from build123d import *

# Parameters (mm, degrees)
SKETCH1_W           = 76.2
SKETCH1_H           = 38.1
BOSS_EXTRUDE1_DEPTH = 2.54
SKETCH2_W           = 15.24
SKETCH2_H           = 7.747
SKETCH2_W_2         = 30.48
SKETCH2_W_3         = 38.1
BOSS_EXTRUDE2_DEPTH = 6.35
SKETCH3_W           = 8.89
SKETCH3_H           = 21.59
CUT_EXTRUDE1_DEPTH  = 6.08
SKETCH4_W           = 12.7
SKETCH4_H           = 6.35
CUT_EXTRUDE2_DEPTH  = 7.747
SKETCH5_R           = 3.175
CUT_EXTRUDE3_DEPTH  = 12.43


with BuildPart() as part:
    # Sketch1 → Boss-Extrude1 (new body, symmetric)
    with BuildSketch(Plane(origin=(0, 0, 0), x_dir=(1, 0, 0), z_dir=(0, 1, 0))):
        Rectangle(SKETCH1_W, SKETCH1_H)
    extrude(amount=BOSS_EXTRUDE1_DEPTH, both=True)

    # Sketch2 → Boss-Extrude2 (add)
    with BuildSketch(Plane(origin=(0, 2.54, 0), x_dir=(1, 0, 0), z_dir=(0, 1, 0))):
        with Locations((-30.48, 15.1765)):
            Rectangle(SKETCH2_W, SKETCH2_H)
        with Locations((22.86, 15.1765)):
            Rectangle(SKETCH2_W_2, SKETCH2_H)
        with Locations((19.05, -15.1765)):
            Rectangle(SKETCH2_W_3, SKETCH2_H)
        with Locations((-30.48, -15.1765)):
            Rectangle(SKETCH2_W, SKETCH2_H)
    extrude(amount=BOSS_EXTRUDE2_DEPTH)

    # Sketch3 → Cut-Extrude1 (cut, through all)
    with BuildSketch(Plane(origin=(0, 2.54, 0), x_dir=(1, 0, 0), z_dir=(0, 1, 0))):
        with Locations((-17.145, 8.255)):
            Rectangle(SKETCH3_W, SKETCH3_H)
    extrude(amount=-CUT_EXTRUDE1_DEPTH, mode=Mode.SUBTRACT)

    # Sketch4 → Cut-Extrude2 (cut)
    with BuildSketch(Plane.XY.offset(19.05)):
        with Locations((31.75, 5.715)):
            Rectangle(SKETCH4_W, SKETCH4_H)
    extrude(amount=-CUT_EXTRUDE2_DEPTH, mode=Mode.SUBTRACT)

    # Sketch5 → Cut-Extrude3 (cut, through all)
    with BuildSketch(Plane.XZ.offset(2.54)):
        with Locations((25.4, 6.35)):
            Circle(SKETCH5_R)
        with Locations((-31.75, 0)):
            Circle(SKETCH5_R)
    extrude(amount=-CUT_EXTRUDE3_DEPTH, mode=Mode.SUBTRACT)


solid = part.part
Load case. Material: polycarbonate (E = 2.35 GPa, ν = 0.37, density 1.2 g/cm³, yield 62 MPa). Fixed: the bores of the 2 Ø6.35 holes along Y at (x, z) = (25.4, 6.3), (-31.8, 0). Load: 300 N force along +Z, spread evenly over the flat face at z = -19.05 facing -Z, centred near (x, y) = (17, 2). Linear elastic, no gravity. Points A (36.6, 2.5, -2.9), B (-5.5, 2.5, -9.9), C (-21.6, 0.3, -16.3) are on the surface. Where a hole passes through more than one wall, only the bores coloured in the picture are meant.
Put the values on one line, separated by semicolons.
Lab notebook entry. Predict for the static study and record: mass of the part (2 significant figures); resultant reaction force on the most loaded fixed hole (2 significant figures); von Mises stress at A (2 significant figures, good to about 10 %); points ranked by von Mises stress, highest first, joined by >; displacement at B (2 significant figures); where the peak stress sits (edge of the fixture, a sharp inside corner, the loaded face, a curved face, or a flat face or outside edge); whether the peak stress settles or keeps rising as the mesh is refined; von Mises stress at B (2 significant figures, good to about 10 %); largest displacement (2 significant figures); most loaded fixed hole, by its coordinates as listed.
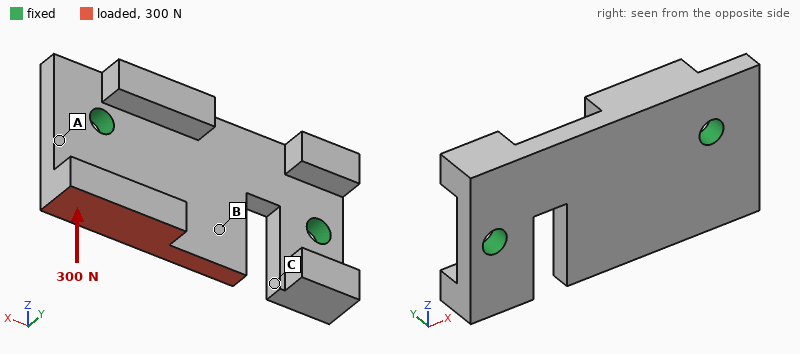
21 g; 250 N; 5.1 MPa; A > B > C; 0.11 mm; edge of the fixture; keeps rising; 2.0 MPa; 0.26 mm; (25.4, 6.3)
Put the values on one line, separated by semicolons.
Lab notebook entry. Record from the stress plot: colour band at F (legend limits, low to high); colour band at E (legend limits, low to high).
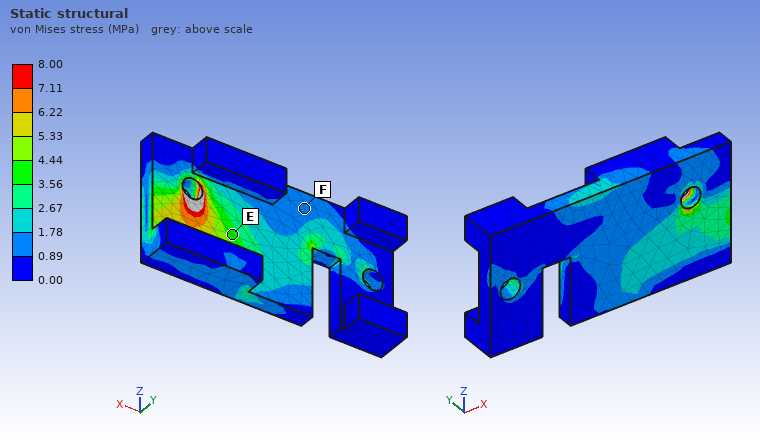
0.89 to 1.78 MPa; 3.56 to 4.44 MPa
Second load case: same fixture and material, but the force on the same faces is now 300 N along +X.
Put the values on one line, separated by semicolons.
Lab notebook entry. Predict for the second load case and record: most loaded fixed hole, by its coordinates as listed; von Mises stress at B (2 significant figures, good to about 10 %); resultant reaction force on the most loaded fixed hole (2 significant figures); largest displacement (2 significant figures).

(25.4, 6.3); 2.9 MPa; 350 N; 0.21 mm
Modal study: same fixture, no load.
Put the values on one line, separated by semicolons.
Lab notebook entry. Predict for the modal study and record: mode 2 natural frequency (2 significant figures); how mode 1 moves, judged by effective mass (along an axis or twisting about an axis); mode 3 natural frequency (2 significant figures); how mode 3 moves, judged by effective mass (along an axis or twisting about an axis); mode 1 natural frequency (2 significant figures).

1700 Hz; along Y; 2100 Hz; along Y; 1100 Hz
